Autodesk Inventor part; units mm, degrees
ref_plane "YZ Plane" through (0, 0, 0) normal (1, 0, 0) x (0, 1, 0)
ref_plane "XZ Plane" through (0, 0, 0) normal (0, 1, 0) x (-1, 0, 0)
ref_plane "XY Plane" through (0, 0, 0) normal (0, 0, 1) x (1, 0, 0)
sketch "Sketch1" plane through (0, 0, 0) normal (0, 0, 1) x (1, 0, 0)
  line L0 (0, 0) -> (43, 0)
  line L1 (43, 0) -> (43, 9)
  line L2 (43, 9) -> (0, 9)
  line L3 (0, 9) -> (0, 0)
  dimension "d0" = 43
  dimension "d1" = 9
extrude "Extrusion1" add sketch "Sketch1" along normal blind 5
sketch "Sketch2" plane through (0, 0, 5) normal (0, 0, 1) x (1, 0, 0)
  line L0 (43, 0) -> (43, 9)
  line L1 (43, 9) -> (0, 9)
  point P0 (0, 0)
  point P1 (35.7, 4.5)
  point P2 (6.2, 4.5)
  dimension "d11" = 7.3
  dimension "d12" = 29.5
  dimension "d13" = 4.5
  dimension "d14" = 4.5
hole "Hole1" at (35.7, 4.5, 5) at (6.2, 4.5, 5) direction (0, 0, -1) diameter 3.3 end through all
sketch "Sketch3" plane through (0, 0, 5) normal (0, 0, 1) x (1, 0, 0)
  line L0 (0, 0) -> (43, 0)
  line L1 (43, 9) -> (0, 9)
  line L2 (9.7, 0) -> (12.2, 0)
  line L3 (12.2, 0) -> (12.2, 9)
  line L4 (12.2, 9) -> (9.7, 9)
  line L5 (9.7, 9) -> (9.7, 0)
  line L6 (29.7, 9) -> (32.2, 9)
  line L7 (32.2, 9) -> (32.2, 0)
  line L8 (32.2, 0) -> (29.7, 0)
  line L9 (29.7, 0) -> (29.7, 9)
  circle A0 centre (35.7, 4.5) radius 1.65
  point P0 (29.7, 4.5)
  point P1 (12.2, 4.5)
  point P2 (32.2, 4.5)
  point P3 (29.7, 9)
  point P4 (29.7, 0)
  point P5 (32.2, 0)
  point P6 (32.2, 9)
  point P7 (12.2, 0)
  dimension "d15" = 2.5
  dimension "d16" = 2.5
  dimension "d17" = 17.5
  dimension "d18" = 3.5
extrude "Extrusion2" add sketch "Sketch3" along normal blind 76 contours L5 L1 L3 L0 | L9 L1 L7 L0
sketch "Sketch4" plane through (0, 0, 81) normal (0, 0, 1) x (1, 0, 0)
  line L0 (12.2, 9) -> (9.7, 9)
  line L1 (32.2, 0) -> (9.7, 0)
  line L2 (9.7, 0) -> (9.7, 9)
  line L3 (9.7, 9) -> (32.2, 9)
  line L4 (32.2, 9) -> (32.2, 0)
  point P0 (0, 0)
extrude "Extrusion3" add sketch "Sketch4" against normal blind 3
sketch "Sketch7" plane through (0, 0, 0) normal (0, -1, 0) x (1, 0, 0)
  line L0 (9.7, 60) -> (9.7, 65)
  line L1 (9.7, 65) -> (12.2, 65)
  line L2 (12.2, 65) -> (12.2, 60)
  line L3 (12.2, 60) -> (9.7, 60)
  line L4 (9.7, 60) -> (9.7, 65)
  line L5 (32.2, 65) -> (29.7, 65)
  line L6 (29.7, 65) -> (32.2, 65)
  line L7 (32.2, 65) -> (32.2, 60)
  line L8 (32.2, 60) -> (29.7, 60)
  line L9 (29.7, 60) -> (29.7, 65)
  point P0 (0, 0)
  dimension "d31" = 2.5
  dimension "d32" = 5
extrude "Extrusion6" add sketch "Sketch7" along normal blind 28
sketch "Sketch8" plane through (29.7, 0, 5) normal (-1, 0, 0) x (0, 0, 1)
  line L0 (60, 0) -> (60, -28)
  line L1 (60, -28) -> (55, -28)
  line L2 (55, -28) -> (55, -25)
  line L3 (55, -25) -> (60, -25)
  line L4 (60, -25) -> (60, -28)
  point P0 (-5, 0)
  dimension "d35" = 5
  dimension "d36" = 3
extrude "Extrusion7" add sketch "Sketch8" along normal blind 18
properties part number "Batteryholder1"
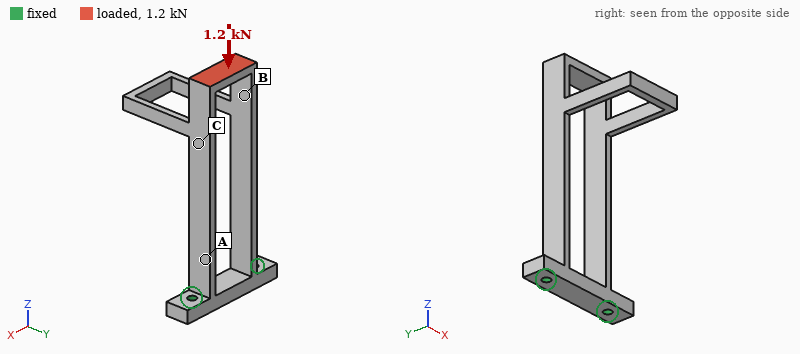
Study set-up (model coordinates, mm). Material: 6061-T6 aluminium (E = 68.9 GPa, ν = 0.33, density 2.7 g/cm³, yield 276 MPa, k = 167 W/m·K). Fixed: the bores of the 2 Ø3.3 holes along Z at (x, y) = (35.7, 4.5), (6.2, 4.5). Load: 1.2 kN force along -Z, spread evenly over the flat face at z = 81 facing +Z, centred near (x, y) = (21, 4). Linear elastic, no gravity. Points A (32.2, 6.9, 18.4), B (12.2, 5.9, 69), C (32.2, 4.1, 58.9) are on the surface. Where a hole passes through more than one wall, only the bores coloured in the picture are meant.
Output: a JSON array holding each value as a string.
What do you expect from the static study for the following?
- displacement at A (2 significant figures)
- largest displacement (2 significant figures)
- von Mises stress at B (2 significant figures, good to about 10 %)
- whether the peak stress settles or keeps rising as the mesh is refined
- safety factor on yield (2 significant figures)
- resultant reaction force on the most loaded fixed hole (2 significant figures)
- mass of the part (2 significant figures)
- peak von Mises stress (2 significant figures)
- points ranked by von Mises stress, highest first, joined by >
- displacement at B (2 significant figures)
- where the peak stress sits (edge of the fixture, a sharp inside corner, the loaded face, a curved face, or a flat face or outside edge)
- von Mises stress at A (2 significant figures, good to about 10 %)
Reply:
["16 µm", "99 µm", "65 MPa", "settles", "1.8", "600 N", "18 g", "150 MPa", "B > A > C", "76 µm", "a flat face or outside edge", "38 MPa"]
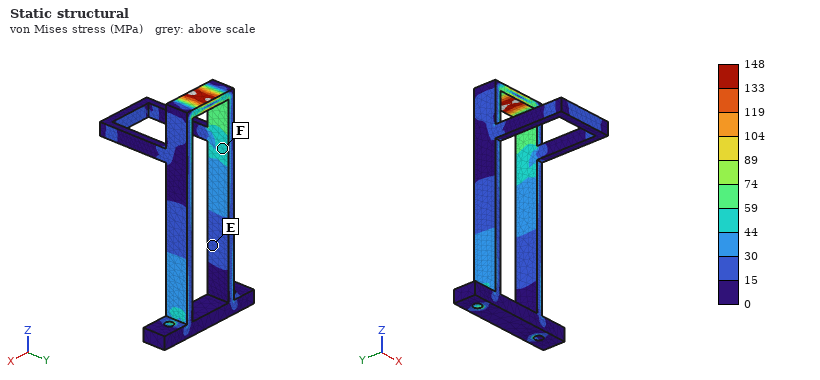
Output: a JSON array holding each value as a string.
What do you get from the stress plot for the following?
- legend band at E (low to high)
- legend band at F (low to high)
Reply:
["15 to 30 MPa", "44 to 59 MPa"]
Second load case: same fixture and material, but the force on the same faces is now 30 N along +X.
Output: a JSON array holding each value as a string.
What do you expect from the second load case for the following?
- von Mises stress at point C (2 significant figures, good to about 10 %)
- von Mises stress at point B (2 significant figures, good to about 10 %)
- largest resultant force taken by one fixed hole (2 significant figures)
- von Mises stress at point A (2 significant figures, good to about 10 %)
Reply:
["27 MPa", "38 MPa", "83 N", "38 MPa"]
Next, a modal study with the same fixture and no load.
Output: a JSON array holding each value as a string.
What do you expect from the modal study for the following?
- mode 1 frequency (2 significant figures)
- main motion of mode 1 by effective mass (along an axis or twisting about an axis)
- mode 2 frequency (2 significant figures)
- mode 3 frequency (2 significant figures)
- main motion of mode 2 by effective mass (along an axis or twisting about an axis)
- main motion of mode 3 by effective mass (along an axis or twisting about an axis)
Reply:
["410 Hz", "along X", "730 Hz", "1000 Hz", "along Y", "twisting about Z"]
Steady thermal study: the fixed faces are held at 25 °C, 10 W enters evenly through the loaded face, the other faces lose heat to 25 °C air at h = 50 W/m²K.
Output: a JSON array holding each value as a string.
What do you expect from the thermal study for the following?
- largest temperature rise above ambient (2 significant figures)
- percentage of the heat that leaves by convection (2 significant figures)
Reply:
["57 K", "64 %"]
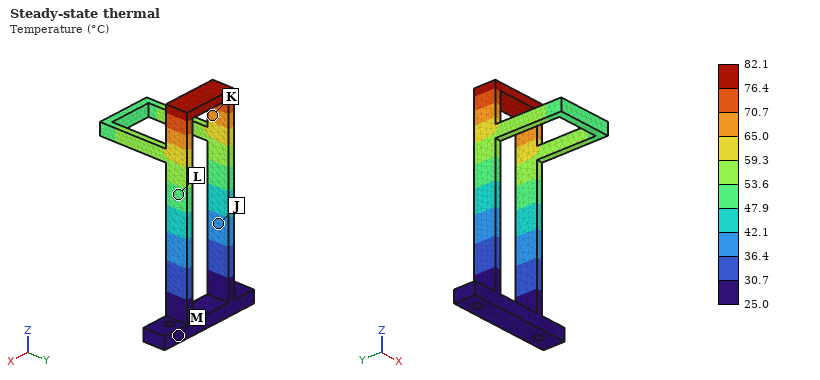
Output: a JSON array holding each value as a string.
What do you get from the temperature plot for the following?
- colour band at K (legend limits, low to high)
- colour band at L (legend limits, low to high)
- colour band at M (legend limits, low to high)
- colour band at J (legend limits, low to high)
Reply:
["65.0 to 70.7 °C", "47.9 to 53.6 °C", "25.0 to 30.7 °C", "36.4 to 42.1 °C"]
